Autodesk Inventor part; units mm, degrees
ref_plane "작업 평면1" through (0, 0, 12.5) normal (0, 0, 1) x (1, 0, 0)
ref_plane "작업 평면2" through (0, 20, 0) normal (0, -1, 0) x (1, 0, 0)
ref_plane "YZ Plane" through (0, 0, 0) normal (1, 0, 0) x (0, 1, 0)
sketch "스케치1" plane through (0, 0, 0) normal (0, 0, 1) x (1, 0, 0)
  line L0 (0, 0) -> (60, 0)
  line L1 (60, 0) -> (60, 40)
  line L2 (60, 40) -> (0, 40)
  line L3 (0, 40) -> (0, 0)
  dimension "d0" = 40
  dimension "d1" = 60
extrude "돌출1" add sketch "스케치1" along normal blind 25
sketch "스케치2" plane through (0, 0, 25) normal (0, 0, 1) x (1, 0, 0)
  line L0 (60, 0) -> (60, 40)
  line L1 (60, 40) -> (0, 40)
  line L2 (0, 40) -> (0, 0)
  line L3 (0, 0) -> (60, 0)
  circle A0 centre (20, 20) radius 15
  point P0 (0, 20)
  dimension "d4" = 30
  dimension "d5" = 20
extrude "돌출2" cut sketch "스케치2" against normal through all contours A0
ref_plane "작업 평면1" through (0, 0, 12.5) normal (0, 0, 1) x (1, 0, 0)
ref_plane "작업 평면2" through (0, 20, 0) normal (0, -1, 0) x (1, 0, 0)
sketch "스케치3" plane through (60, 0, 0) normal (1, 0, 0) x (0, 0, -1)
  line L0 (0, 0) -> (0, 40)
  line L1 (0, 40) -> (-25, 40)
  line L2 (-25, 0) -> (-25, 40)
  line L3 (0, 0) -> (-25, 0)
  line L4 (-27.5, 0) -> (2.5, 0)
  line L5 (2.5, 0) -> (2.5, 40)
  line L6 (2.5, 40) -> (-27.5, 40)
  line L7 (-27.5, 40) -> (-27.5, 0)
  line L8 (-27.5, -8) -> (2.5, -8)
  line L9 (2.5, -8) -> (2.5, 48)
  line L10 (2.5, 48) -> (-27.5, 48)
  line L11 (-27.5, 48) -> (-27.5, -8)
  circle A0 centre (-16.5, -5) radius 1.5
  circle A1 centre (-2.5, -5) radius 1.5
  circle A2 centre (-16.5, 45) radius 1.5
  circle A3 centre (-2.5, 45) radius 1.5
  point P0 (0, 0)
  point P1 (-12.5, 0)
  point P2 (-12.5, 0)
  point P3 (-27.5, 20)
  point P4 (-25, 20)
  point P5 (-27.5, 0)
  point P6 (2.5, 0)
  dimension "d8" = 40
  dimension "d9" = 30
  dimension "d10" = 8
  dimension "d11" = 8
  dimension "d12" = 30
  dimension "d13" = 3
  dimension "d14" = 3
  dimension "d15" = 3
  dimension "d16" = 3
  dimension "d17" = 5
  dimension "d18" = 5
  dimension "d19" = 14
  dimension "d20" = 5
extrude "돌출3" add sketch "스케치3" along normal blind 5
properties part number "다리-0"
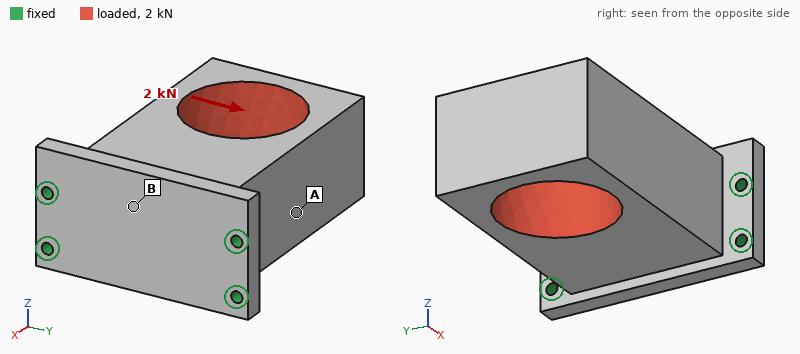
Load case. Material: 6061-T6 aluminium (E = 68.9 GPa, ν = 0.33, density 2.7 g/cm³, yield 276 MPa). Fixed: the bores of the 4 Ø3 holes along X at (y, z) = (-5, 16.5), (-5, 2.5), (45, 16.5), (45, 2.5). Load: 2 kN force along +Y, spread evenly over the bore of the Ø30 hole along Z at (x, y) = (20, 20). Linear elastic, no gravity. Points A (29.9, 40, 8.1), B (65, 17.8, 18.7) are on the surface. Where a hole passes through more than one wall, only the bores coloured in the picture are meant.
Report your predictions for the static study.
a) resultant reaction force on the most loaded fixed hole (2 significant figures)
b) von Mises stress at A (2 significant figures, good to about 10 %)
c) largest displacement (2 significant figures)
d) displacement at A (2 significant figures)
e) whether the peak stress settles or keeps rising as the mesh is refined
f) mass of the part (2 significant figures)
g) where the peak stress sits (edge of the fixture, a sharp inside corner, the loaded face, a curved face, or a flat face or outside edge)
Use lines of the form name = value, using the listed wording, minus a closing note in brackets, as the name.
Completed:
resultant reaction force on the most loaded fixed hole = 1.2 kN
von Mises stress at A = 21 MPa
largest displacement = 64 µm
displacement at A = 26 µm
whether the peak stress settles or keeps rising as the mesh is refined = keeps rising
mass of the part = 140 g
where the peak stress sits = edge of the fixture
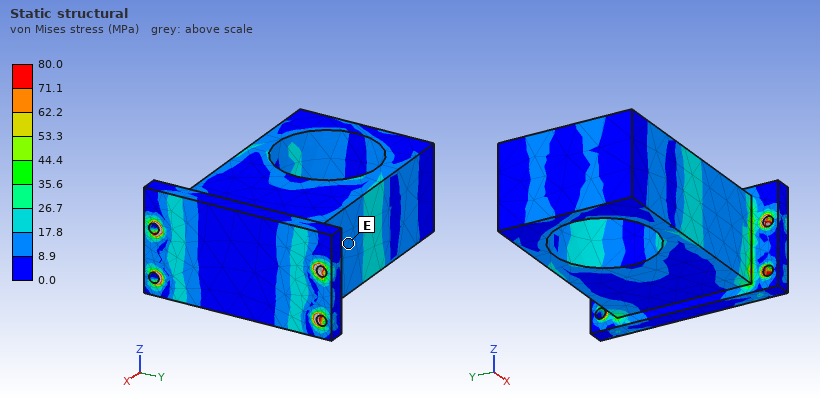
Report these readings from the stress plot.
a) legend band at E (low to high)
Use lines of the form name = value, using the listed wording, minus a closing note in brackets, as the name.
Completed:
legend band at E = 8.9 to 17.8 MPa
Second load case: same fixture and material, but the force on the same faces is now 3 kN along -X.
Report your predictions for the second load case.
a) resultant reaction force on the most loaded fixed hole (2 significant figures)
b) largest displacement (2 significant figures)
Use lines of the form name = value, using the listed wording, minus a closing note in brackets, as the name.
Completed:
resultant reaction force on the most loaded fixed hole = 1.1 kN
largest displacement = 26 µm
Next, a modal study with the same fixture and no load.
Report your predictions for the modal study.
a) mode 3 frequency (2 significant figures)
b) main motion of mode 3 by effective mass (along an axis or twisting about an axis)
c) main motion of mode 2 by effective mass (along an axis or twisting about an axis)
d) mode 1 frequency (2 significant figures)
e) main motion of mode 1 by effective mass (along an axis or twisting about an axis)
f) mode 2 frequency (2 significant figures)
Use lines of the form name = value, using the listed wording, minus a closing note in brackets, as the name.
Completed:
mode 3 frequency = 7900 Hz
main motion of mode 3 by effective mass = twisting about X
main motion of mode 2 by effective mass = along Y
mode 1 frequency = 2000 Hz
main motion of mode 1 by effective mass = along Z
mode 2 frequency = 4000 Hz
